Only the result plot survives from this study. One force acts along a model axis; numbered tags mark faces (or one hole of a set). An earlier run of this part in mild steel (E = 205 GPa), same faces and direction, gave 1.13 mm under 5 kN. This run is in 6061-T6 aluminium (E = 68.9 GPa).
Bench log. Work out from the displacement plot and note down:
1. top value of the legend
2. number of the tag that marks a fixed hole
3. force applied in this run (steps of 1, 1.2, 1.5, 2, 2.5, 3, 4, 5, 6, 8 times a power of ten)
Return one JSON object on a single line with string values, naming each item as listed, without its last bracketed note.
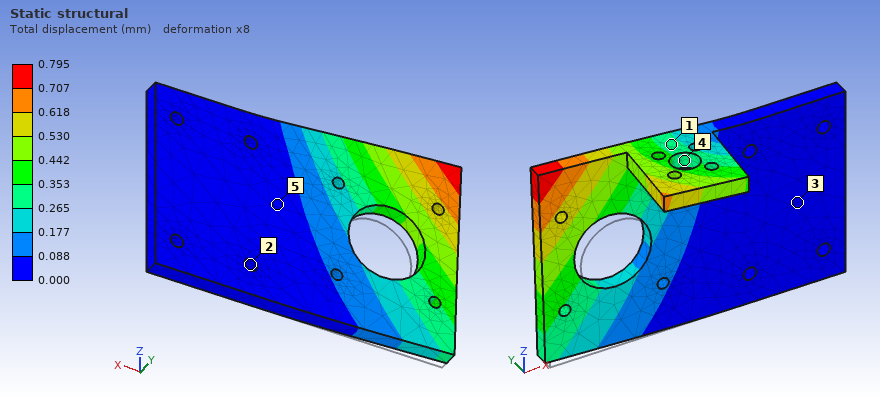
{"top value of the legend": "0.795 mm", "number of the tag that marks a fixed hole": "2", "force applied in this run": "1.2 kN"}
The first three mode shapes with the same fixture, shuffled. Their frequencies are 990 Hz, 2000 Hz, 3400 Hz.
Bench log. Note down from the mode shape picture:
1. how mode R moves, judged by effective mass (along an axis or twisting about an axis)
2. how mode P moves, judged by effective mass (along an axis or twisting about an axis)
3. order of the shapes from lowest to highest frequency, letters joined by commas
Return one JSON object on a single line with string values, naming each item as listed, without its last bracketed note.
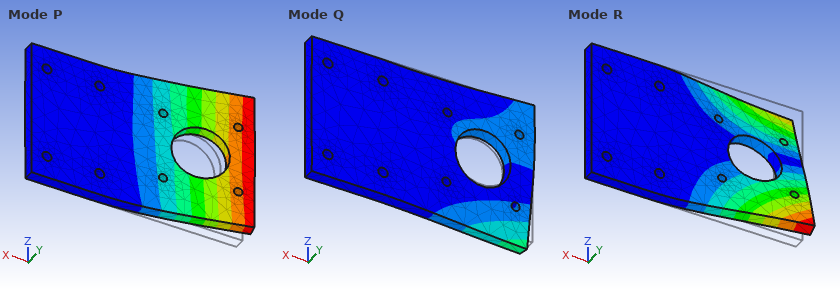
{"how mode R moves, judged by effective mass": "twisting about X", "how mode P moves, judged by effective mass": "along Y", "order of the shapes from lowest to highest frequency, letters joined by commas": "P, R, Q"}
